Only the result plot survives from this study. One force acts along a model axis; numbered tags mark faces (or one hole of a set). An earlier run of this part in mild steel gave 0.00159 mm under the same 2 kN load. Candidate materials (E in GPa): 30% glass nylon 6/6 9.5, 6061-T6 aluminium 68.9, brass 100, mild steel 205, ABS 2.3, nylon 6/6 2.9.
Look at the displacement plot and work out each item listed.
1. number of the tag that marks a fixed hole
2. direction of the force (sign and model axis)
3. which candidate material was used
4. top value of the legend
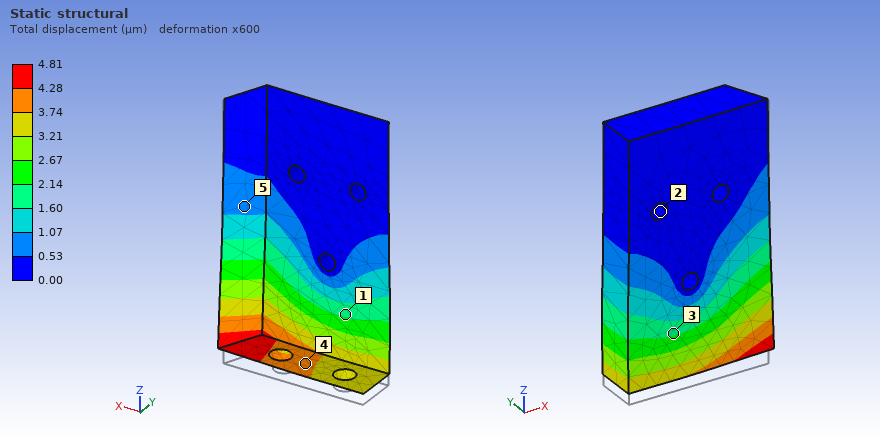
2
+Z
6061-T6 aluminium
4.81 µm
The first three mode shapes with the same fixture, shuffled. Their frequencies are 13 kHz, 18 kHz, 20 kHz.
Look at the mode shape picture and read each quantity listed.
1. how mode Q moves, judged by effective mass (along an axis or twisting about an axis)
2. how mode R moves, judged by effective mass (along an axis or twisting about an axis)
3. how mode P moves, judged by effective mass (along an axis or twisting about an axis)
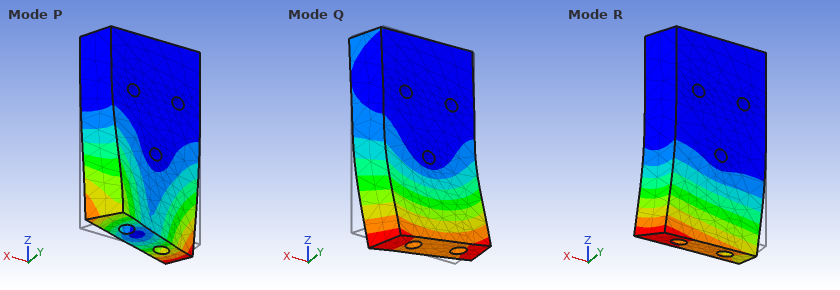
along X
along Y
twisting about Z
